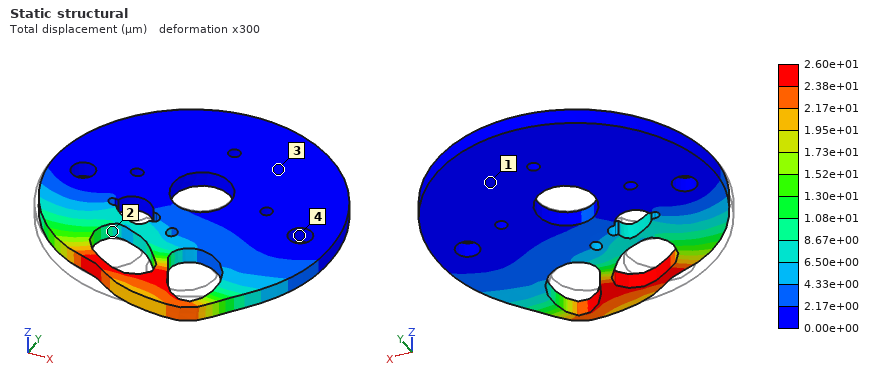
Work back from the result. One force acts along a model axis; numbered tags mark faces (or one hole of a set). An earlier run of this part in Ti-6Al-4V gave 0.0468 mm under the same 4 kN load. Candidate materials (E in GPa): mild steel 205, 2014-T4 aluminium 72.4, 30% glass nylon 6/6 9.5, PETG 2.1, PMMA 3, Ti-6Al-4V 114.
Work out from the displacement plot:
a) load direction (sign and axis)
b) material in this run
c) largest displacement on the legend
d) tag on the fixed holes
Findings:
+X
mild steel
2.60e+01 µm
4
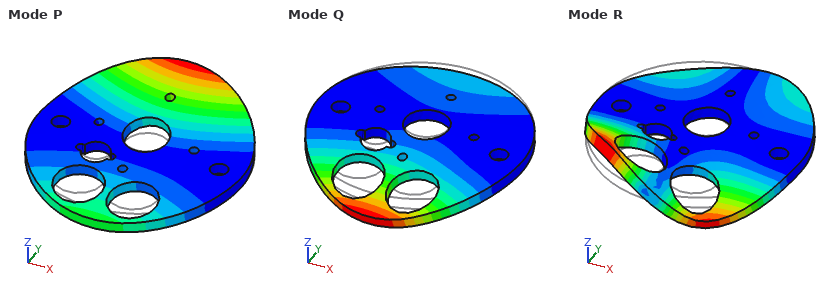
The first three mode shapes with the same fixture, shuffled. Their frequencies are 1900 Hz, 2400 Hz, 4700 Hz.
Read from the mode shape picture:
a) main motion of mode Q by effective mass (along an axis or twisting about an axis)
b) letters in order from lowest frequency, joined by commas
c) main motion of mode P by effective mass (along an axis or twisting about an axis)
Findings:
along Z
P, Q, R
along Z
